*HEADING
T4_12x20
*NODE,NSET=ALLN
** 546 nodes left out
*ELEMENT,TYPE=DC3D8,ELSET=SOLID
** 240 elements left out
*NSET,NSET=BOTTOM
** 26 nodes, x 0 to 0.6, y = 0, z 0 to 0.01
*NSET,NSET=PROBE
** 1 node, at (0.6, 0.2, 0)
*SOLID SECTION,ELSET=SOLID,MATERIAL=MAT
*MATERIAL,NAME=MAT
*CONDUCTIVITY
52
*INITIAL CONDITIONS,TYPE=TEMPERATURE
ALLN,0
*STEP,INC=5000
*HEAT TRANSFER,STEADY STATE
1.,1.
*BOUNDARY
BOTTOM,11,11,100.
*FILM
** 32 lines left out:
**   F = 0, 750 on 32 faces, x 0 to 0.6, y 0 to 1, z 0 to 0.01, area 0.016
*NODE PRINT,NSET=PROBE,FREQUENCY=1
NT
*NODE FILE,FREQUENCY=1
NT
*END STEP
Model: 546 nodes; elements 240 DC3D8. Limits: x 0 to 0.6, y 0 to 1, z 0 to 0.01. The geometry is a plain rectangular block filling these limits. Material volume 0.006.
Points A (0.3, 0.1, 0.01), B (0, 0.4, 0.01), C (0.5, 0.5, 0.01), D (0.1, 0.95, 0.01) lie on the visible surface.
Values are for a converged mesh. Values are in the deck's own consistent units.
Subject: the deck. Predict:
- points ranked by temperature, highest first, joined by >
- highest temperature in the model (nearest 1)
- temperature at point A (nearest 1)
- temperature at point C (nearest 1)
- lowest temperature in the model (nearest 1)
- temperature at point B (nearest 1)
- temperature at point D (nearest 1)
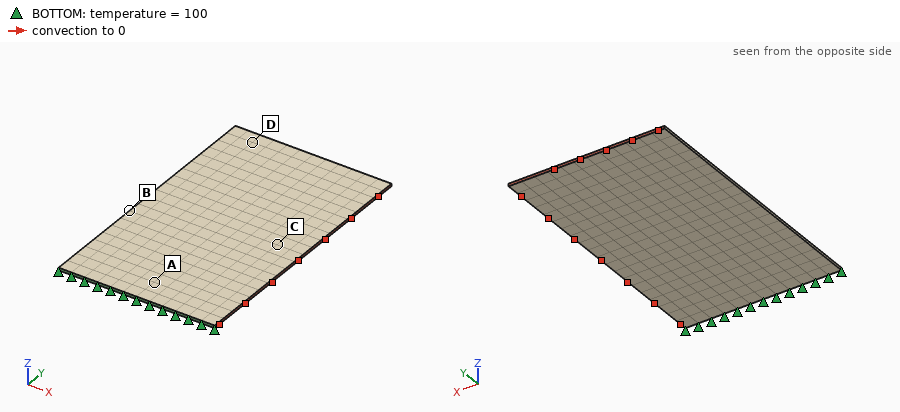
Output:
A > B > C > D
100
80
15
1
45
6
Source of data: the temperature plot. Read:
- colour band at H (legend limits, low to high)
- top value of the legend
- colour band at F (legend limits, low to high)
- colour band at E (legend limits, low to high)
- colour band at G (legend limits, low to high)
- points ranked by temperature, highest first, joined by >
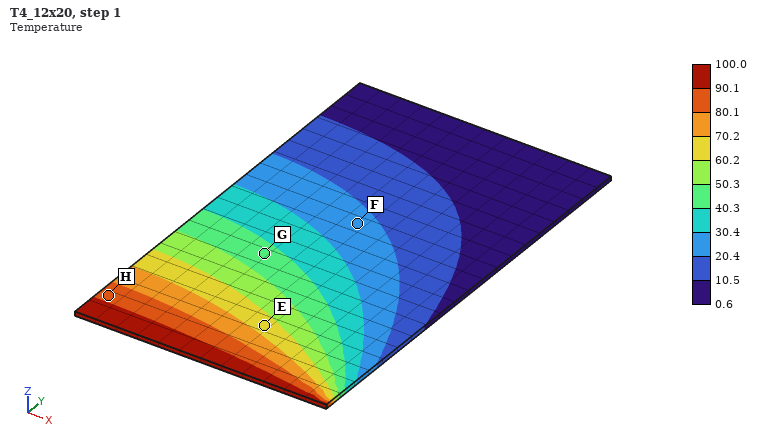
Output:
80.1 to 90.1
100.0
20.4 to 30.4
60.2 to 70.2
40.3 to 50.3
H > E > G > F
